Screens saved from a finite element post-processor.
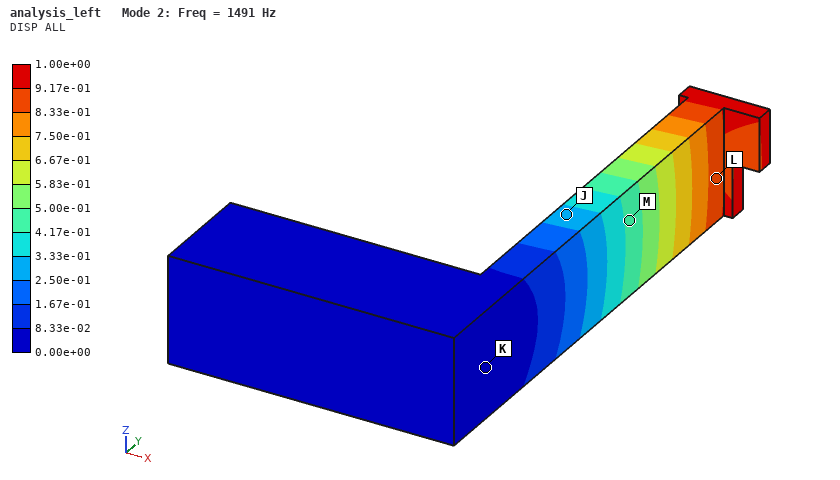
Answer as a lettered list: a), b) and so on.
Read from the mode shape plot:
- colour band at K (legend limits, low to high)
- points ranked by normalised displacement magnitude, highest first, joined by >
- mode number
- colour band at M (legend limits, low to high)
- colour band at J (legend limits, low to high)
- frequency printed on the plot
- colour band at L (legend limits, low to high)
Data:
a) 0.00e+00 to 8.33e-02
b) L > M > J > K
c) 2
d) 4.17e-01 to 5.00e-01
e) 2.50e-01 to 3.33e-01
f) 1491 Hz
g) 8.33e-01 to 9.17e-01
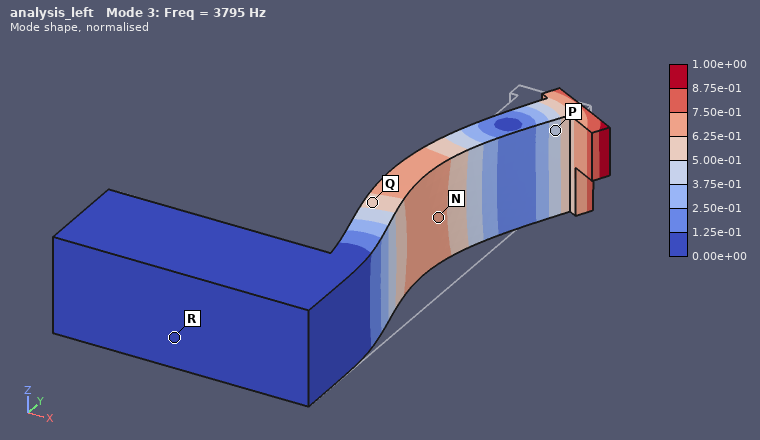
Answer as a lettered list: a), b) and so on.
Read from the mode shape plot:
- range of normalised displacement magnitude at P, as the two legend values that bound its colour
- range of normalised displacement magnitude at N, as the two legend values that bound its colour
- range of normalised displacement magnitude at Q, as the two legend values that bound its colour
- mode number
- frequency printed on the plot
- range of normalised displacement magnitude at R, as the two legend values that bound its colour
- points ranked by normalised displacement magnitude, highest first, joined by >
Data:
a) 3.75e-01 to 5.00e-01
b) 6.25e-01 to 7.50e-01
c) 5.00e-01 to 6.25e-01
d) 3
e) 3795 Hz
f) 0.00e+00 to 1.25e-01
g) N > Q > P > R
